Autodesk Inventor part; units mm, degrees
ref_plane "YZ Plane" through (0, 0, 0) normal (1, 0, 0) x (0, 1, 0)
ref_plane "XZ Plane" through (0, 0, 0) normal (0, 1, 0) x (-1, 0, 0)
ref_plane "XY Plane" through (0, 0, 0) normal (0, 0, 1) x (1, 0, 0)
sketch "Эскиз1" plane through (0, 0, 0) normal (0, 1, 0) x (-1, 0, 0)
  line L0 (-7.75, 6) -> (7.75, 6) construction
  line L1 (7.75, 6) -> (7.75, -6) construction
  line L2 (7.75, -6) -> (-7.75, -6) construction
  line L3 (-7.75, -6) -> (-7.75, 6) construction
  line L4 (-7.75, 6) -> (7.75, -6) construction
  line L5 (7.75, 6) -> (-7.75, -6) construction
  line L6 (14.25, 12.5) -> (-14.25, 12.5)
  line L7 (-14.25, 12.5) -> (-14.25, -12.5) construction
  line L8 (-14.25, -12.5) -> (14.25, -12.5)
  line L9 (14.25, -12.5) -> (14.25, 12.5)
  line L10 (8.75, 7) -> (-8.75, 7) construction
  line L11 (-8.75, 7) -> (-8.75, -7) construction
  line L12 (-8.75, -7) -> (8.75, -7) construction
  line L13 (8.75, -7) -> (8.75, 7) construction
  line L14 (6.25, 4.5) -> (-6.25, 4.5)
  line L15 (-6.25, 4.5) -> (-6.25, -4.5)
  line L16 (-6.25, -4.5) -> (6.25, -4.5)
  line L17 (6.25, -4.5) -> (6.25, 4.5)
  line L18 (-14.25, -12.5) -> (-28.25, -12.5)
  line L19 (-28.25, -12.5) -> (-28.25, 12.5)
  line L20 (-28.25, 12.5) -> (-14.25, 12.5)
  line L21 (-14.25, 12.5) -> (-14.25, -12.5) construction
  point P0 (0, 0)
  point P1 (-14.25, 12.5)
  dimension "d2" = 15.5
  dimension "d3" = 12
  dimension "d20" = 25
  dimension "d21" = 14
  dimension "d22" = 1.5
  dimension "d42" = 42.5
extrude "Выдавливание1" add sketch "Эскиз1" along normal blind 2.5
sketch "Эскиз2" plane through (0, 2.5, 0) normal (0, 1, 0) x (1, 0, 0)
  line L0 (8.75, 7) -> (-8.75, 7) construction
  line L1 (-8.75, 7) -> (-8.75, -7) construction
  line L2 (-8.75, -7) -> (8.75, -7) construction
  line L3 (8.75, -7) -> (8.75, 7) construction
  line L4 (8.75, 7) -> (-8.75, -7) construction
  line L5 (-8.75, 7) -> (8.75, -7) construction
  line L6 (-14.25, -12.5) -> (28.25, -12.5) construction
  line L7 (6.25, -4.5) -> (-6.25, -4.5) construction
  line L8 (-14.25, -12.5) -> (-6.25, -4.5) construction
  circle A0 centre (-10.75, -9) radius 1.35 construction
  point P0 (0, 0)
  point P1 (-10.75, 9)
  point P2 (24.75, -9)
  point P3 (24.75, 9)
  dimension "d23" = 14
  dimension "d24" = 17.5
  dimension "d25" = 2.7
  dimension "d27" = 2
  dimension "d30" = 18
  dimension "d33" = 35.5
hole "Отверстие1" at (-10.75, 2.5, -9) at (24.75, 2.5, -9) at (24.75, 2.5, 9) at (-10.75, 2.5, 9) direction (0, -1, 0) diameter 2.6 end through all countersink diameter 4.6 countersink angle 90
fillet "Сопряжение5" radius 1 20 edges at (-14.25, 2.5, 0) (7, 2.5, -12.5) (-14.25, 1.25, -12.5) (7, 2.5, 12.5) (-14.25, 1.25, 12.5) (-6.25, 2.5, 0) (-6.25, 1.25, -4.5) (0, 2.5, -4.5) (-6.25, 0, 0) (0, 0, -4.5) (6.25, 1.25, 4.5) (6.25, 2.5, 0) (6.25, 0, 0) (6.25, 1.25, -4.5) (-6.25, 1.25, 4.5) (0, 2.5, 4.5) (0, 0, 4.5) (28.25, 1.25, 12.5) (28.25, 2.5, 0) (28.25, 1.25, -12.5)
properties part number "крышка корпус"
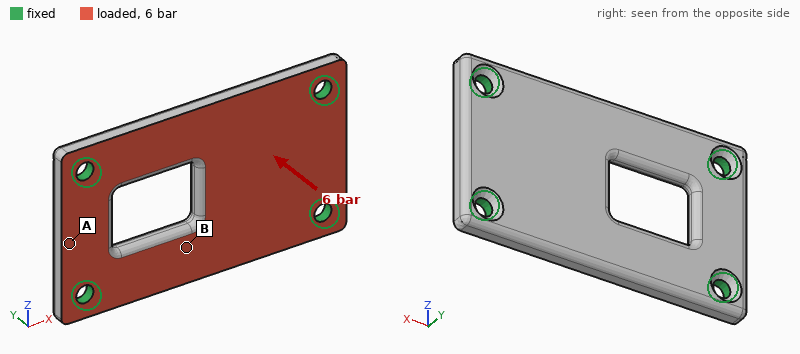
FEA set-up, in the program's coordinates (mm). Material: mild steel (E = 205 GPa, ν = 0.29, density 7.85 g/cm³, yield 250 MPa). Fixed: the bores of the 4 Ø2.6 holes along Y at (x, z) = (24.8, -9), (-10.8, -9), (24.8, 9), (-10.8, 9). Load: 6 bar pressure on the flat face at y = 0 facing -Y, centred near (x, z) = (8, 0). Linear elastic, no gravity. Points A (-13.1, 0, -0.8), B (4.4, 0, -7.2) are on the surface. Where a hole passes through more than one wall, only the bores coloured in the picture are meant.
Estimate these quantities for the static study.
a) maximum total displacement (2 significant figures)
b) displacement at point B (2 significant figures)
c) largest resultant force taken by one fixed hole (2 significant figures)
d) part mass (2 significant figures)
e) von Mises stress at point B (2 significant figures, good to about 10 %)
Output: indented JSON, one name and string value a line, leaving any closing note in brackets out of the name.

{
  "maximum total displacement": "14 µm",
  "displacement at point B": "12 µm",
  "largest resultant force taken by one fixed hole": "160 N",
  "part mass": "18 g",
  "von Mises stress at point B": "34 MPa"
}
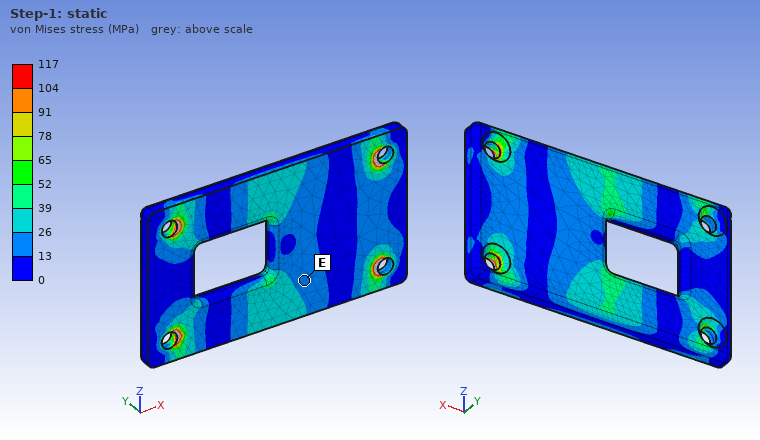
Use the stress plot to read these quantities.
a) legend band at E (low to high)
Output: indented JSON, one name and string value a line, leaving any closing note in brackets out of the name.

{
  "legend band at E": "13 to 26 MPa"
}
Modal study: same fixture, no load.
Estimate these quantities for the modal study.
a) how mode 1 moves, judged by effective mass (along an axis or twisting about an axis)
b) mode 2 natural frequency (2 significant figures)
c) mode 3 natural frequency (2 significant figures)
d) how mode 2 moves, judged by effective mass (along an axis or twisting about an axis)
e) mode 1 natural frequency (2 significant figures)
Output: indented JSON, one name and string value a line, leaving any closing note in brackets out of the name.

{
  "how mode 1 moves, judged by effective mass": "along Y",
  "mode 2 natural frequency": "12 kHz",
  "mode 3 natural frequency": "23 kHz",
  "how mode 2 moves, judged by effective mass": "twisting about X",
  "mode 1 natural frequency": "8700 Hz"
}
